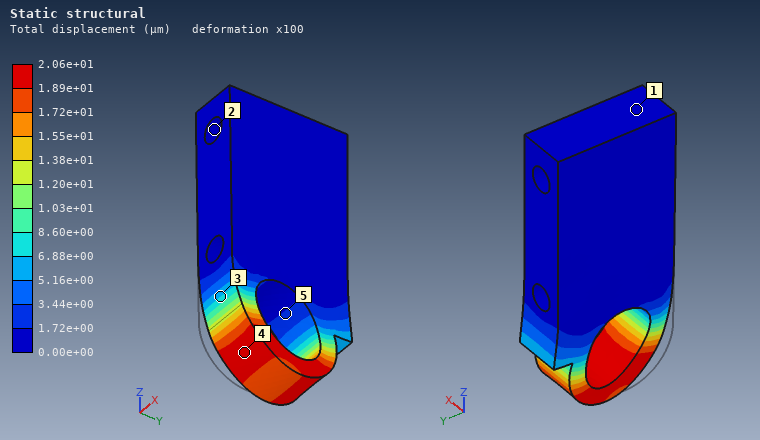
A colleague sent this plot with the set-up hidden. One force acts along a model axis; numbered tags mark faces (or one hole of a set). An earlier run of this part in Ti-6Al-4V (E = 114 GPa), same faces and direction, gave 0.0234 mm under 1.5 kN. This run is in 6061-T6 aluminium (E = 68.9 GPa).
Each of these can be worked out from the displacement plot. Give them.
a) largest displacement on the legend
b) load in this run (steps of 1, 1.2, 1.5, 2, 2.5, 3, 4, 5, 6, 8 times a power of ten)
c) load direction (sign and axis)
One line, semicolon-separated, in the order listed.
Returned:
2.06e+01 µm; 800 N; +Y
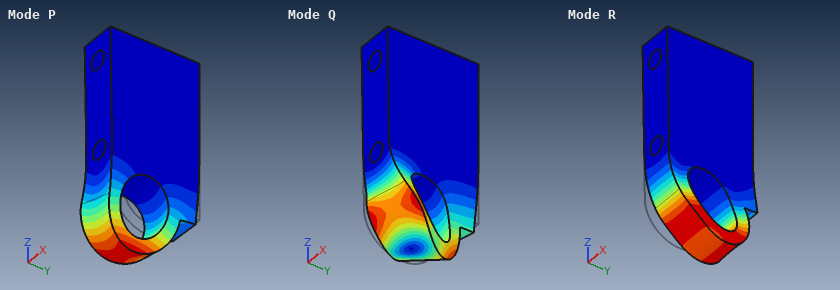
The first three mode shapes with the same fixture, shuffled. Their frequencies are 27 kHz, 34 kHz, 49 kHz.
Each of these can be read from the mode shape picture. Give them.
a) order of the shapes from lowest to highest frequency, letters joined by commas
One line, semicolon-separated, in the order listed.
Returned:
P, R, Q
